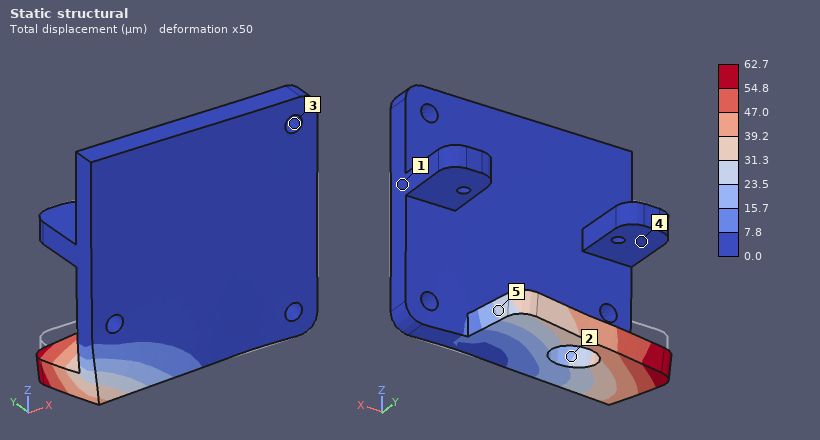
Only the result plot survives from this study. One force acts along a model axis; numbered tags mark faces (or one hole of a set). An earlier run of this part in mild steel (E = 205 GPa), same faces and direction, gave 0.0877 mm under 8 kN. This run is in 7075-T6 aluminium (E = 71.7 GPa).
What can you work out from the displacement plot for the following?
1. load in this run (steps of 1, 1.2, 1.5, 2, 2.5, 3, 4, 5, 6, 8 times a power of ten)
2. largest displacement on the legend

2 kN
62.7 µm
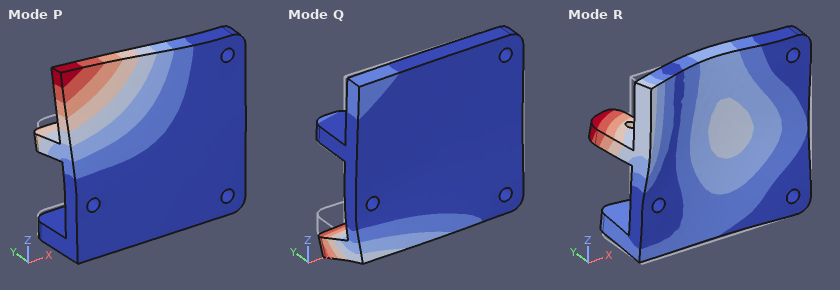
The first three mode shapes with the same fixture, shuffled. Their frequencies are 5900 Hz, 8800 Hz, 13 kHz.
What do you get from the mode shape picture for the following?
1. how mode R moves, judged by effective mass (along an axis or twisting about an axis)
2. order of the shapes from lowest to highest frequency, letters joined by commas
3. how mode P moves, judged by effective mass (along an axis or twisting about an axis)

along Y
P, Q, R
along Y
